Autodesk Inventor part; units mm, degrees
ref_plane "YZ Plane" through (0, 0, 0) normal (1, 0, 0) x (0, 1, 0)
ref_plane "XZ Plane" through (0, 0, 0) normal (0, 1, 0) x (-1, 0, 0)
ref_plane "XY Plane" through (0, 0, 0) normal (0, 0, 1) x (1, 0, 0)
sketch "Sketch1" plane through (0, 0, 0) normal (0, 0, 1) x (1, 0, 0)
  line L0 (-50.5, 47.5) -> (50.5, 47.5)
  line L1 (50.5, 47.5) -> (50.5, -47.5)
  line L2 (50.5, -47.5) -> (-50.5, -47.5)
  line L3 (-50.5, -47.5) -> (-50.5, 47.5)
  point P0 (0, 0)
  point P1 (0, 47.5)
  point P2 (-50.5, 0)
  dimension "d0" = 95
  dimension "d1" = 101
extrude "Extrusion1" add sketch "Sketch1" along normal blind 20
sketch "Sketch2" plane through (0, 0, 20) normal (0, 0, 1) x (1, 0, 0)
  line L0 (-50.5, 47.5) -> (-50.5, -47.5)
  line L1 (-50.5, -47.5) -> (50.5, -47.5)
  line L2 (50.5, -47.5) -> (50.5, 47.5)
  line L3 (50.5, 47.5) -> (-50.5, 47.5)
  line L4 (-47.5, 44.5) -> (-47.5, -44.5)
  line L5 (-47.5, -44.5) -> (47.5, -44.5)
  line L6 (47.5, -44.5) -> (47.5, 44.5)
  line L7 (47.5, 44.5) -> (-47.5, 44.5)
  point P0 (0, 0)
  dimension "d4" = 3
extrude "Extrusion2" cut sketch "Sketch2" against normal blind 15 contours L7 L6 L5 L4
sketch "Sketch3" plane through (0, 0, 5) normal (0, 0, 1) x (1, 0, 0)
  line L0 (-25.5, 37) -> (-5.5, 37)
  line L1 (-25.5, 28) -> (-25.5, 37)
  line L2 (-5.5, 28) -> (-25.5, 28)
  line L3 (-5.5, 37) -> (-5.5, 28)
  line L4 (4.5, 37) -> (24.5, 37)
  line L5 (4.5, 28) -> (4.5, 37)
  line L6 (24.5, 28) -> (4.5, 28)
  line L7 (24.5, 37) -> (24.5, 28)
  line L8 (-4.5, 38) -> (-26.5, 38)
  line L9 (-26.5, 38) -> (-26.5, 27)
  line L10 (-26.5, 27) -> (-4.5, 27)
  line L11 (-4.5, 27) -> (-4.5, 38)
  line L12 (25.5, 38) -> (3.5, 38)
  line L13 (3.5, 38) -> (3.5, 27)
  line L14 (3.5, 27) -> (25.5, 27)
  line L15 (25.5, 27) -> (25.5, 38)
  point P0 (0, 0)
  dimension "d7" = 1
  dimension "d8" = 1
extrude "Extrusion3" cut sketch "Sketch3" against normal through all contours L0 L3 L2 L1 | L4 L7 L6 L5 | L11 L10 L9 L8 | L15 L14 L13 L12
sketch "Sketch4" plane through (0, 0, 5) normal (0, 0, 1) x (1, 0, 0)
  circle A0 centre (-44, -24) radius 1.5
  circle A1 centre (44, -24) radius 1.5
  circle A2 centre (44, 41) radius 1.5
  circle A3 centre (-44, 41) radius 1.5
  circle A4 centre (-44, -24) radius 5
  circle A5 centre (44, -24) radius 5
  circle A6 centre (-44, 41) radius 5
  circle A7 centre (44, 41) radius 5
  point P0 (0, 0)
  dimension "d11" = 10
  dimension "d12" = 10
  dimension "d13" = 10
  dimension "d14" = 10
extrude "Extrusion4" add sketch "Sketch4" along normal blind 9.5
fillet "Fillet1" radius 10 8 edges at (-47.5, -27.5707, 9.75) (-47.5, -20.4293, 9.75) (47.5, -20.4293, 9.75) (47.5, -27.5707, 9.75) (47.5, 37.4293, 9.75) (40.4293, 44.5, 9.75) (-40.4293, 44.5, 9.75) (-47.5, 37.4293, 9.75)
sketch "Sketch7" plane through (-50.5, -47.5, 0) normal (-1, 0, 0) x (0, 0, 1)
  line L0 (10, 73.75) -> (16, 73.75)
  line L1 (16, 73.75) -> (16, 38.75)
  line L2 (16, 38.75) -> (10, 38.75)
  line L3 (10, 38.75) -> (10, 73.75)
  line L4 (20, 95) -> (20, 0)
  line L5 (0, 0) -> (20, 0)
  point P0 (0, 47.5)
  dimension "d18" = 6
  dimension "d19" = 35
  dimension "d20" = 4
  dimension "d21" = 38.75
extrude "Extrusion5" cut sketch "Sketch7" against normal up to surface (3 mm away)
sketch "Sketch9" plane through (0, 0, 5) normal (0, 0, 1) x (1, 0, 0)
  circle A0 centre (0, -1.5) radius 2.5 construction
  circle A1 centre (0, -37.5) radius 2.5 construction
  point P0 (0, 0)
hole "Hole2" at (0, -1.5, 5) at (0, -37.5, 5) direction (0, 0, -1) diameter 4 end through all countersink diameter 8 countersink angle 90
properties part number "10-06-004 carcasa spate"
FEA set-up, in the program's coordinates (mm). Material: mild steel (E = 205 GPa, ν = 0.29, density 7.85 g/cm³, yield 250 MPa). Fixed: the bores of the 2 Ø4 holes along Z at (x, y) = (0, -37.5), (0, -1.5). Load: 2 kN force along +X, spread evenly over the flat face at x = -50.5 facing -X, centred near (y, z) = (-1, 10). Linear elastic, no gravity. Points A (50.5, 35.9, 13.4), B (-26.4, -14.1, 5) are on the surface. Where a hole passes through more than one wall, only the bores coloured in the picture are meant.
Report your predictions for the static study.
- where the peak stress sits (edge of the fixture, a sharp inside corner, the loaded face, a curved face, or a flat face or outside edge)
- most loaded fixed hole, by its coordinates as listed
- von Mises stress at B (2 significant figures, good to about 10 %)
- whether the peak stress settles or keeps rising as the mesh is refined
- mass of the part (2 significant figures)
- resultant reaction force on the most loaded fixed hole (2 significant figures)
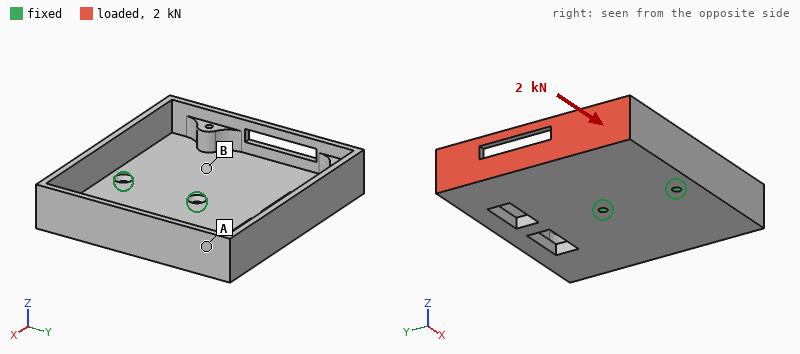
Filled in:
edge of the fixture
(0, -1.5)
20 MPa
keeps rising
510 g
2.0 kN
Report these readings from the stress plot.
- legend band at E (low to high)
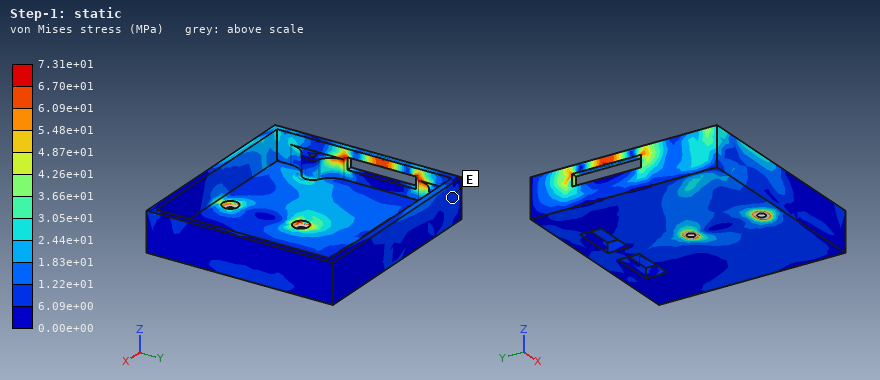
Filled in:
6.09e+00 to 1.22e+01 MPa
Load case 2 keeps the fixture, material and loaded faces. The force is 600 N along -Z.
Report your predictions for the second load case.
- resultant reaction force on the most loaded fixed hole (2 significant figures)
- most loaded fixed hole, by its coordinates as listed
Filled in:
570 N
(0, -1.5)
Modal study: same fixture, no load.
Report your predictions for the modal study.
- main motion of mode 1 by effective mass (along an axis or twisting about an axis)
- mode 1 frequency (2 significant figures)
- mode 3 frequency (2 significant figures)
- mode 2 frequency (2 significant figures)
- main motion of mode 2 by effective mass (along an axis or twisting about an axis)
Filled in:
twisting about Y
660 Hz
1500 Hz
1000 Hz
along Z
